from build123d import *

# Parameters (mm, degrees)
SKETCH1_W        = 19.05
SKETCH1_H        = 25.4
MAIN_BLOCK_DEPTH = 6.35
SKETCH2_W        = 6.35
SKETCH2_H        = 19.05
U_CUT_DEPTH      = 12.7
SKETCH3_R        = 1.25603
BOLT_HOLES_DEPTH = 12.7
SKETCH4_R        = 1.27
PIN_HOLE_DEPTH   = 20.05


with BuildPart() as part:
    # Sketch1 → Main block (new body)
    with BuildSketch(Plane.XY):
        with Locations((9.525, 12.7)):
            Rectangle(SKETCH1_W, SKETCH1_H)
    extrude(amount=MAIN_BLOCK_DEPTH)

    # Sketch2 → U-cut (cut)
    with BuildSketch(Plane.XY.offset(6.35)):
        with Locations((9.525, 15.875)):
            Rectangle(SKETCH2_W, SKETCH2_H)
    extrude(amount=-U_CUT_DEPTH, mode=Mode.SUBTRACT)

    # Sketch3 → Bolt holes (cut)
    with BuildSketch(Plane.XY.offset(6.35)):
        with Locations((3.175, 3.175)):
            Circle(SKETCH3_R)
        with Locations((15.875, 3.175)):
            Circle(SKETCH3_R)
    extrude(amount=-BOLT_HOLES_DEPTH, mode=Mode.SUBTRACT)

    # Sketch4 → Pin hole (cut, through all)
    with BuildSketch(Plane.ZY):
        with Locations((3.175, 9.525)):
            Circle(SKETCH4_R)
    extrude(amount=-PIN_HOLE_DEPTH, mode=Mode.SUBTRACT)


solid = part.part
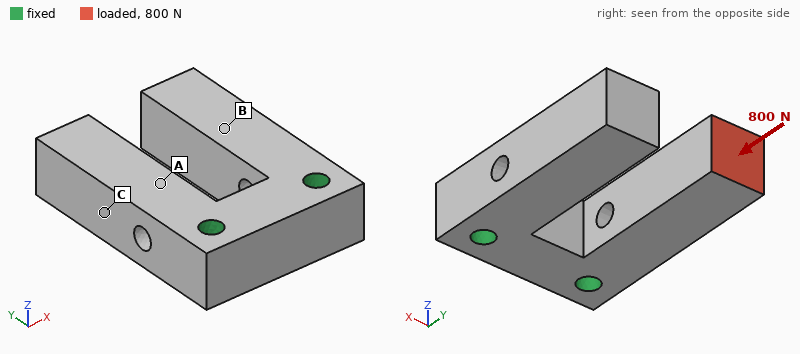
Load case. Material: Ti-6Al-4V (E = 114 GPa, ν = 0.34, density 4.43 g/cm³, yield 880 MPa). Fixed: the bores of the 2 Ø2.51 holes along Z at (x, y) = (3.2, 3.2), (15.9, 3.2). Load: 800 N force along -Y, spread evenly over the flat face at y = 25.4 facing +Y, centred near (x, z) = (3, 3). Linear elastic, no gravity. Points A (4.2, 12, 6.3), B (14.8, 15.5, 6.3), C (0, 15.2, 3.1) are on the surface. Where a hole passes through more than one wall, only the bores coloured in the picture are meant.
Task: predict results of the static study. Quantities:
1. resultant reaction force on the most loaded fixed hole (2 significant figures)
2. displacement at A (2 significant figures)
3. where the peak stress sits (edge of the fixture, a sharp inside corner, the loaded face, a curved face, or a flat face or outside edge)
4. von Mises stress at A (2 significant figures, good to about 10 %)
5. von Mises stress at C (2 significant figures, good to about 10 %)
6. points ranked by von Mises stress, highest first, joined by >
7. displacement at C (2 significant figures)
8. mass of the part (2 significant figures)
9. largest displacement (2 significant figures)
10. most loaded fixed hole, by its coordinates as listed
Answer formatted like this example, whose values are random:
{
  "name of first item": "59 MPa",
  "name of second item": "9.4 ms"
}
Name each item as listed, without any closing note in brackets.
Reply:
{
  "resultant reaction force on the most loaded fixed hole": "780 N",
  "displacement at A": "1.8 µm",
  "where the peak stress sits": "a curved face",
  "von Mises stress at A": "28 MPa",
  "von Mises stress at C": "18 MPa",
  "points ranked by von Mises stress, highest first, joined by >": "A > C > B",
  "displacement at C": "2.8 µm",
  "mass of the part": "9.6 g",
  "largest displacement": "4.7 µm",
  "most loaded fixed hole, by its coordinates as listed": "(3.2, 3.2)"
}
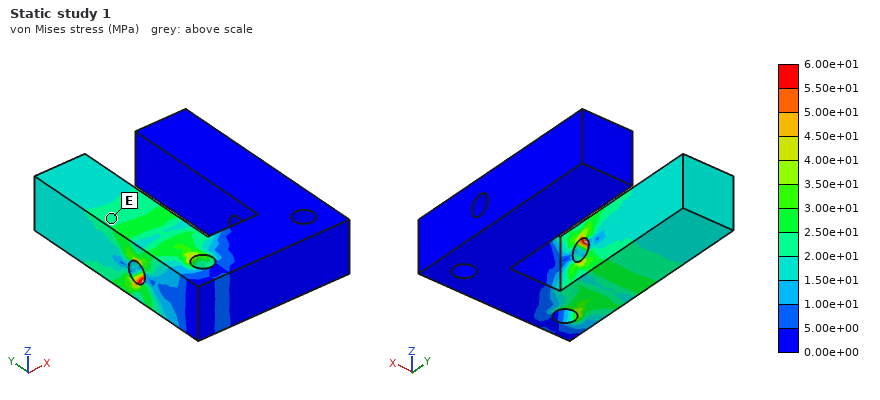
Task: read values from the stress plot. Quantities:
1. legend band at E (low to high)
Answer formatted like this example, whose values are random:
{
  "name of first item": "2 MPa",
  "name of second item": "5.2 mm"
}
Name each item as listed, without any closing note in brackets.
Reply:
{
  "legend band at E": "2.00e+01 to 2.50e+01 MPa"
}
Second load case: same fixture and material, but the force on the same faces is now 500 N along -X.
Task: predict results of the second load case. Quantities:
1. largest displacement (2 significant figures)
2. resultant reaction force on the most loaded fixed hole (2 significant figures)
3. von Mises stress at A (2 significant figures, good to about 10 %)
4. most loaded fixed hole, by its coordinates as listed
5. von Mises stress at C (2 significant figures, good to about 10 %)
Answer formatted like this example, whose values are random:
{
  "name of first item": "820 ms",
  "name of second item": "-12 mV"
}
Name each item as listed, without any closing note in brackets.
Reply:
{
  "largest displacement": "0.15 mm",
  "resultant reaction force on the most loaded fixed hole": "640 N",
  "von Mises stress at A": "100 MPa",
  "most loaded fixed hole, by its coordinates as listed": "(15.9, 3.2)",
  "von Mises stress at C": "110 MPa"
}
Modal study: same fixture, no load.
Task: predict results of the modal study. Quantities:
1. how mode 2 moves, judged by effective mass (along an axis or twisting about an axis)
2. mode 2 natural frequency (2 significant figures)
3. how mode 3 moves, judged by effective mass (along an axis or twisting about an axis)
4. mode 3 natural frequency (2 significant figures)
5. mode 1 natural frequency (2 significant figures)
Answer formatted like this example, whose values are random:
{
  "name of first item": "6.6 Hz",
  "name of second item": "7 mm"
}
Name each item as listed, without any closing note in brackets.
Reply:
{
  "how mode 2 moves, judged by effective mass": "along X",
  "mode 2 natural frequency": "9400 Hz",
  "how mode 3 moves, judged by effective mass": "along Z",
  "mode 3 natural frequency": "10 kHz",
  "mode 1 natural frequency": "9100 Hz"
}
